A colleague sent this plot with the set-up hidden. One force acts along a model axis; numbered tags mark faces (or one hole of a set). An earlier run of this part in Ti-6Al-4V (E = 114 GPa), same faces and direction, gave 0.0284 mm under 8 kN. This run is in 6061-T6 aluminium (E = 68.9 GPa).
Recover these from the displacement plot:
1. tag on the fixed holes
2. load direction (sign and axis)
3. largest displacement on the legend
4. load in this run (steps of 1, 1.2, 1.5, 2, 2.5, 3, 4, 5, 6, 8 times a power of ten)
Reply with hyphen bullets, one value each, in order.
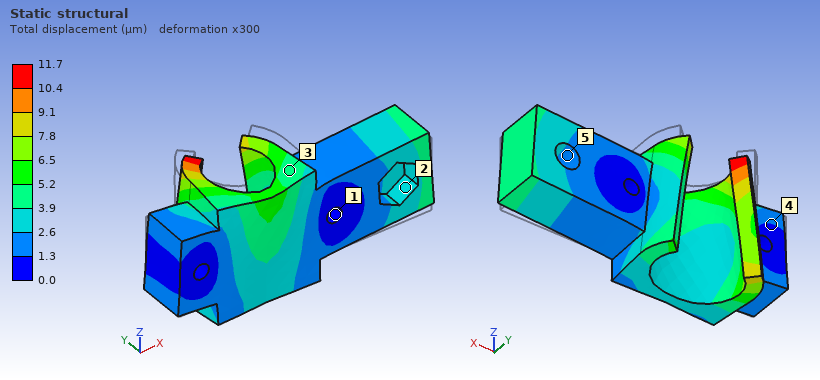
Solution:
- 1
- -Z
- 11.7 µm
- 2 kN
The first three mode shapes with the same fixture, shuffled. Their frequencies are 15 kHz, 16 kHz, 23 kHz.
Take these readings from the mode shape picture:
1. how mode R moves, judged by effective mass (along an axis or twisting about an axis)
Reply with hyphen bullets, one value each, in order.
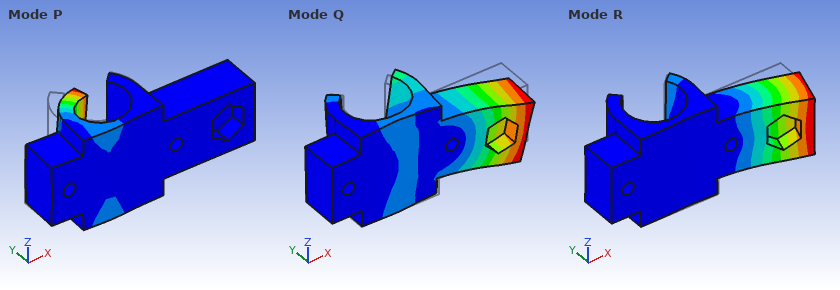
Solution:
- along Y
